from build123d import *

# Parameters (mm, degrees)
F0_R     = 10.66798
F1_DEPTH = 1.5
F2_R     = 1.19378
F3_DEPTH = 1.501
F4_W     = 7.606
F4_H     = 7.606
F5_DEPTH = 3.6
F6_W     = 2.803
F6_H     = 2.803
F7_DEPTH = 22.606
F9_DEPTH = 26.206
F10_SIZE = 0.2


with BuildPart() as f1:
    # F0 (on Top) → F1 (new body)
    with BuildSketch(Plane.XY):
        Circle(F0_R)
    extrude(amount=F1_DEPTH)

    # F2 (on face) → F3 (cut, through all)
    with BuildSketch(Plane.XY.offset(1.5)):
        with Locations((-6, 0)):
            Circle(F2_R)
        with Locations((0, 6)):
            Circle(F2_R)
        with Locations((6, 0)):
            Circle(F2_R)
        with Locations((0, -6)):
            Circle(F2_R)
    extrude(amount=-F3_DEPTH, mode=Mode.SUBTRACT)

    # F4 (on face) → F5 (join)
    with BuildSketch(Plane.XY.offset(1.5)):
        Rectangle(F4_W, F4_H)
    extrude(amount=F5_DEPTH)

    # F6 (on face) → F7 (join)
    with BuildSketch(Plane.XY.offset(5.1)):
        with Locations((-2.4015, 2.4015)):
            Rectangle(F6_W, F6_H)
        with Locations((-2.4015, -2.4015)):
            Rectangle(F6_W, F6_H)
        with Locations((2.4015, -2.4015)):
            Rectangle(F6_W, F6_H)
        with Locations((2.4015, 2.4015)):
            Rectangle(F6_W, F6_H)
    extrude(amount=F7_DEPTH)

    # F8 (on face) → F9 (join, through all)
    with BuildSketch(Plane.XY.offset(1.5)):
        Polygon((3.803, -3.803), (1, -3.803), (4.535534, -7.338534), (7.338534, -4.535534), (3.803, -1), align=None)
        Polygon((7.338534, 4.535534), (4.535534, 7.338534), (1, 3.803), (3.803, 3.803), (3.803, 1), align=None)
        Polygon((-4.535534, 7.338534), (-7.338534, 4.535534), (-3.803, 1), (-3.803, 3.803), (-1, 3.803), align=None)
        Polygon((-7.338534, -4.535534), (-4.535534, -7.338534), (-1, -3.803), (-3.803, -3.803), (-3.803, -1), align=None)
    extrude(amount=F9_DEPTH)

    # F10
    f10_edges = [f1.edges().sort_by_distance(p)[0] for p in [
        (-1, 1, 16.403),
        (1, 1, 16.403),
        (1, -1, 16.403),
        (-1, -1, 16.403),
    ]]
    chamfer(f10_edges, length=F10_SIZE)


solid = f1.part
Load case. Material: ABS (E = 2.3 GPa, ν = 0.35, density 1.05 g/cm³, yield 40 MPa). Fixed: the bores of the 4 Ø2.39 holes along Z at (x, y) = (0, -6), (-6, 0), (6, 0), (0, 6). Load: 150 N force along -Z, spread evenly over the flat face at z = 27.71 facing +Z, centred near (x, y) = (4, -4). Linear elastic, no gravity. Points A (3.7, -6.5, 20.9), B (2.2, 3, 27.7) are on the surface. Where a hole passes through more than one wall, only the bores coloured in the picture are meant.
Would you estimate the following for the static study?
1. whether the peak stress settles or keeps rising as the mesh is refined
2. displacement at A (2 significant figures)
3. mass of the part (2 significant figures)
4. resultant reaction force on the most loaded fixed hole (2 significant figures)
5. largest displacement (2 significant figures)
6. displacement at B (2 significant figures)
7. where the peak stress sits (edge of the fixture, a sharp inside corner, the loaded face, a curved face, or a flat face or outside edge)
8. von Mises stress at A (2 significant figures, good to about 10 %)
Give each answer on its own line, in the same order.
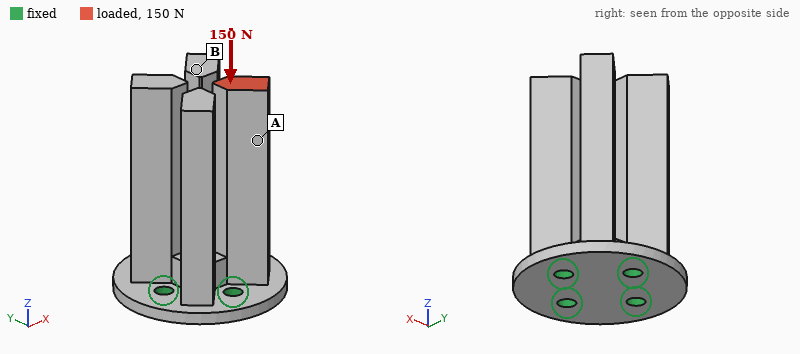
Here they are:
keeps rising
0.19 mm
3.2 g
85 N
0.25 mm
0.080 mm
edge of the fixture
6.3 MPa
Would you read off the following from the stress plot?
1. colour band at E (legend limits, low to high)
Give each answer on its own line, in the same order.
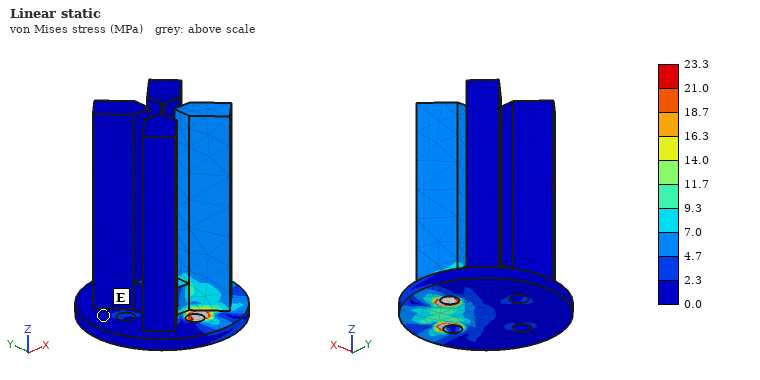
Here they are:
0.0 to 2.3 MPa
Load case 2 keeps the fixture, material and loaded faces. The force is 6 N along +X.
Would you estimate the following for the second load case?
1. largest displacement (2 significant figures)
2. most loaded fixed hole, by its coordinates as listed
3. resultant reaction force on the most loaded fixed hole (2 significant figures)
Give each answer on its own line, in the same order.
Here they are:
0.42 mm
(6, 0)
17 N
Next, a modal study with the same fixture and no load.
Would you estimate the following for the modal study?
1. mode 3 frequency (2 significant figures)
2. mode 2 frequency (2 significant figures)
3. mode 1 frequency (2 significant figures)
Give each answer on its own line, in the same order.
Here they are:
1300 Hz
1300 Hz
1300 Hz
